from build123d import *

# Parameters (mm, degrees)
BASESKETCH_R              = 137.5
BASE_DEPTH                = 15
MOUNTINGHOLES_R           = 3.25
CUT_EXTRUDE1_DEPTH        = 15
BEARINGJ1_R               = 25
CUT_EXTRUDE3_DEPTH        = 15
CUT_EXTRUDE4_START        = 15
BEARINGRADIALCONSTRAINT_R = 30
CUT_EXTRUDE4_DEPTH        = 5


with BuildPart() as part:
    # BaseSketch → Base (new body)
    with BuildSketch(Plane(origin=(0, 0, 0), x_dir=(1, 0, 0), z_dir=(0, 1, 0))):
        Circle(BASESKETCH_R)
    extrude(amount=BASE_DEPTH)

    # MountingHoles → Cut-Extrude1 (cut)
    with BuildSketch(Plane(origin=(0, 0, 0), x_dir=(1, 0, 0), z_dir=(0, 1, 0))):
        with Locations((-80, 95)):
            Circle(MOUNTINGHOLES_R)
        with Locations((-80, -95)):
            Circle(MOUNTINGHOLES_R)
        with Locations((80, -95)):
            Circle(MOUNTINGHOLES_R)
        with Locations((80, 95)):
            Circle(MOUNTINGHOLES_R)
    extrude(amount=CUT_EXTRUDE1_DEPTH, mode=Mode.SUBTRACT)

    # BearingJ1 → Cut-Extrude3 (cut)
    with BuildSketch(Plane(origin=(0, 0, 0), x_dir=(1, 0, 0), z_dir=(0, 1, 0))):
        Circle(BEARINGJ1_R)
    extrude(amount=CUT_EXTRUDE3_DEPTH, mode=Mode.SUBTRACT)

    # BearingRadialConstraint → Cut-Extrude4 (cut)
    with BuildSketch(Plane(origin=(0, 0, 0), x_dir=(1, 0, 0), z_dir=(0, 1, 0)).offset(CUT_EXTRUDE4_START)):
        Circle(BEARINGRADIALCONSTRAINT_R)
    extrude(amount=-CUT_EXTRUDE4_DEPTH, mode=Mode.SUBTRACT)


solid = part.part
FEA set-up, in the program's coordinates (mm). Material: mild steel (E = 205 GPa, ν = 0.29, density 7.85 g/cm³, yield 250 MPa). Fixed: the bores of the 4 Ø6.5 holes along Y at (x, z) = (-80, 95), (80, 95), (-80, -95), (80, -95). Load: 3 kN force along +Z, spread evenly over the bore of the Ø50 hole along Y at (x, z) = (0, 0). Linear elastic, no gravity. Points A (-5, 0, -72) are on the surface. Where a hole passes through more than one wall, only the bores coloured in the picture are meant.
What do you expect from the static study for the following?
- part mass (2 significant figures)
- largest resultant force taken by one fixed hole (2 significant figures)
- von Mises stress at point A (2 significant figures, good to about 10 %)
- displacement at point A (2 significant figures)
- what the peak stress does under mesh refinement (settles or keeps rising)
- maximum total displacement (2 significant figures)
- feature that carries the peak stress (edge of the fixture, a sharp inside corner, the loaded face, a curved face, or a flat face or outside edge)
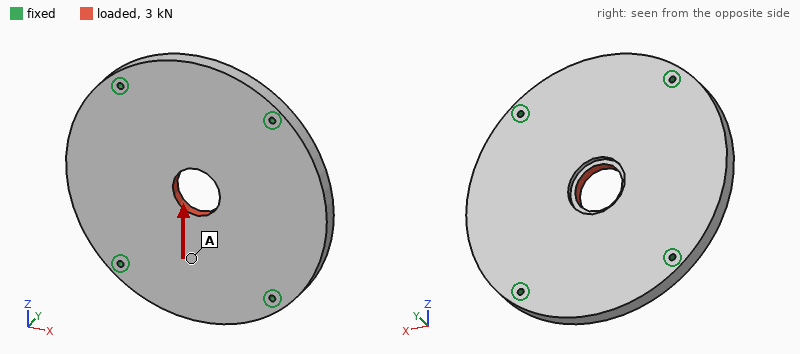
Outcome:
6.7 kg
770 N
0.58 MPa
0.52 µm
keeps rising
0.80 µm
edge of the fixture
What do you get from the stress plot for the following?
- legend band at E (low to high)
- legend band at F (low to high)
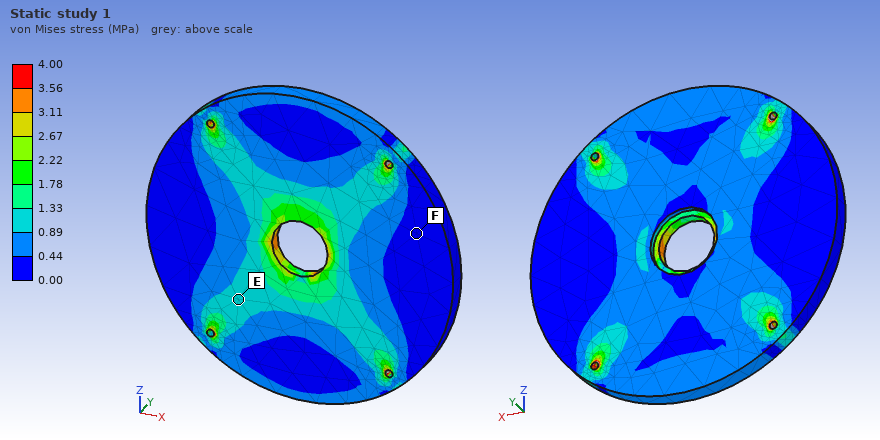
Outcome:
0.89 to 1.33 MPa
0.00 to 0.44 MPa
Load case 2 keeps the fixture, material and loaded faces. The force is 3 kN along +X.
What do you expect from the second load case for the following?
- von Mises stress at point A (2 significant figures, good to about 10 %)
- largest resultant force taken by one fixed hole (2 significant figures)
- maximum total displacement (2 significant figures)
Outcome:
0.77 MPa
770 N
0.90 µm
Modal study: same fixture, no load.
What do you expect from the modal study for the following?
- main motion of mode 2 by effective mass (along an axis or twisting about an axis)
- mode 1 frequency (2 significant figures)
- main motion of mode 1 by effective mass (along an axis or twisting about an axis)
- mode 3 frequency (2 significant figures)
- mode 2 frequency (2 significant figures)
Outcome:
twisting about Z
1400 Hz
along Y
1800 Hz
1600 Hz
